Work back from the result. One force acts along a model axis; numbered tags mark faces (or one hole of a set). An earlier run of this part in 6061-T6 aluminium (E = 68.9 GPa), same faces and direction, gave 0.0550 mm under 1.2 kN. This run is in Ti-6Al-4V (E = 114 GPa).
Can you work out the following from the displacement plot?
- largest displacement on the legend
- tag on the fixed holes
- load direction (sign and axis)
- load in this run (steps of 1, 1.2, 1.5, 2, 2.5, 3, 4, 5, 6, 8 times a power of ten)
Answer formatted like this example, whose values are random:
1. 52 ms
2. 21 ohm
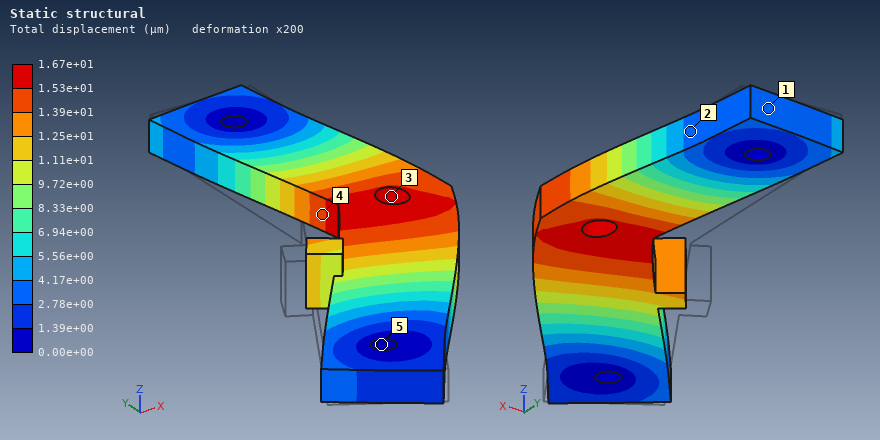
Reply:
1. 1.67e+01 µm
2. 5
3. +X
4. 600 N
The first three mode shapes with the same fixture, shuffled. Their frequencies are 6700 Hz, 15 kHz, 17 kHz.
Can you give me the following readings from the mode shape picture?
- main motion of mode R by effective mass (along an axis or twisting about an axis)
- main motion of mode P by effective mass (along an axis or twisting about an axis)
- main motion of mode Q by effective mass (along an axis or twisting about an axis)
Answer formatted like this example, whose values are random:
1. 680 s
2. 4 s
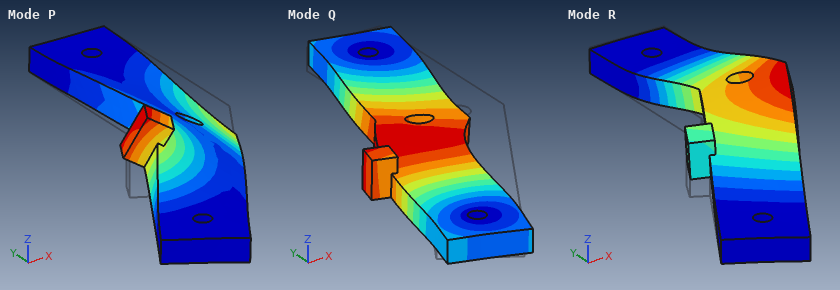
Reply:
1. along Z
2. twisting about Y
3. along X
